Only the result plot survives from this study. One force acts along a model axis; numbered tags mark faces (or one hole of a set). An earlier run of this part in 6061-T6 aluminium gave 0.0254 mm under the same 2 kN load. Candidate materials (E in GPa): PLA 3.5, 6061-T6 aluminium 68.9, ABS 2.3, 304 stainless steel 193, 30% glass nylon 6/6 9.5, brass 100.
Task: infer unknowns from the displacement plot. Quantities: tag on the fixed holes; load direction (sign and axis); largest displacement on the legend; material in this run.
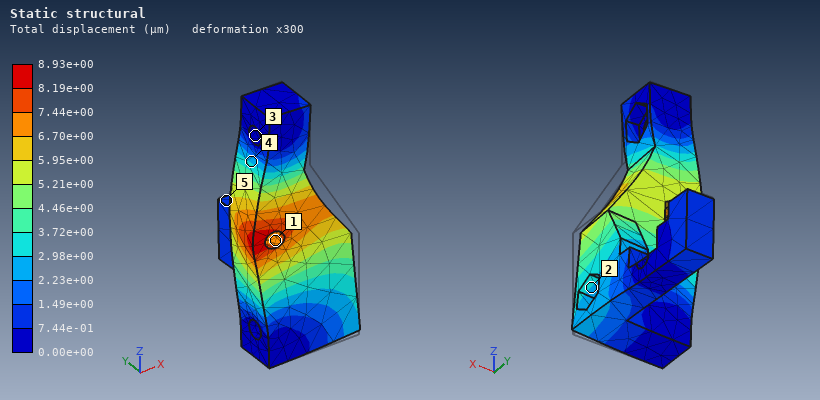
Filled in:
3
-X
8.93e+00 µm
304 stainless steel
